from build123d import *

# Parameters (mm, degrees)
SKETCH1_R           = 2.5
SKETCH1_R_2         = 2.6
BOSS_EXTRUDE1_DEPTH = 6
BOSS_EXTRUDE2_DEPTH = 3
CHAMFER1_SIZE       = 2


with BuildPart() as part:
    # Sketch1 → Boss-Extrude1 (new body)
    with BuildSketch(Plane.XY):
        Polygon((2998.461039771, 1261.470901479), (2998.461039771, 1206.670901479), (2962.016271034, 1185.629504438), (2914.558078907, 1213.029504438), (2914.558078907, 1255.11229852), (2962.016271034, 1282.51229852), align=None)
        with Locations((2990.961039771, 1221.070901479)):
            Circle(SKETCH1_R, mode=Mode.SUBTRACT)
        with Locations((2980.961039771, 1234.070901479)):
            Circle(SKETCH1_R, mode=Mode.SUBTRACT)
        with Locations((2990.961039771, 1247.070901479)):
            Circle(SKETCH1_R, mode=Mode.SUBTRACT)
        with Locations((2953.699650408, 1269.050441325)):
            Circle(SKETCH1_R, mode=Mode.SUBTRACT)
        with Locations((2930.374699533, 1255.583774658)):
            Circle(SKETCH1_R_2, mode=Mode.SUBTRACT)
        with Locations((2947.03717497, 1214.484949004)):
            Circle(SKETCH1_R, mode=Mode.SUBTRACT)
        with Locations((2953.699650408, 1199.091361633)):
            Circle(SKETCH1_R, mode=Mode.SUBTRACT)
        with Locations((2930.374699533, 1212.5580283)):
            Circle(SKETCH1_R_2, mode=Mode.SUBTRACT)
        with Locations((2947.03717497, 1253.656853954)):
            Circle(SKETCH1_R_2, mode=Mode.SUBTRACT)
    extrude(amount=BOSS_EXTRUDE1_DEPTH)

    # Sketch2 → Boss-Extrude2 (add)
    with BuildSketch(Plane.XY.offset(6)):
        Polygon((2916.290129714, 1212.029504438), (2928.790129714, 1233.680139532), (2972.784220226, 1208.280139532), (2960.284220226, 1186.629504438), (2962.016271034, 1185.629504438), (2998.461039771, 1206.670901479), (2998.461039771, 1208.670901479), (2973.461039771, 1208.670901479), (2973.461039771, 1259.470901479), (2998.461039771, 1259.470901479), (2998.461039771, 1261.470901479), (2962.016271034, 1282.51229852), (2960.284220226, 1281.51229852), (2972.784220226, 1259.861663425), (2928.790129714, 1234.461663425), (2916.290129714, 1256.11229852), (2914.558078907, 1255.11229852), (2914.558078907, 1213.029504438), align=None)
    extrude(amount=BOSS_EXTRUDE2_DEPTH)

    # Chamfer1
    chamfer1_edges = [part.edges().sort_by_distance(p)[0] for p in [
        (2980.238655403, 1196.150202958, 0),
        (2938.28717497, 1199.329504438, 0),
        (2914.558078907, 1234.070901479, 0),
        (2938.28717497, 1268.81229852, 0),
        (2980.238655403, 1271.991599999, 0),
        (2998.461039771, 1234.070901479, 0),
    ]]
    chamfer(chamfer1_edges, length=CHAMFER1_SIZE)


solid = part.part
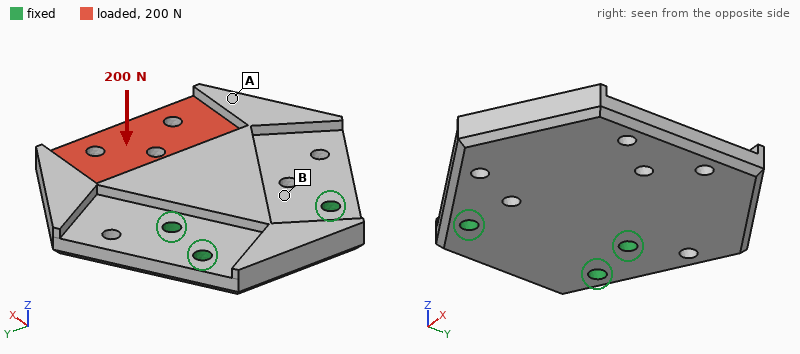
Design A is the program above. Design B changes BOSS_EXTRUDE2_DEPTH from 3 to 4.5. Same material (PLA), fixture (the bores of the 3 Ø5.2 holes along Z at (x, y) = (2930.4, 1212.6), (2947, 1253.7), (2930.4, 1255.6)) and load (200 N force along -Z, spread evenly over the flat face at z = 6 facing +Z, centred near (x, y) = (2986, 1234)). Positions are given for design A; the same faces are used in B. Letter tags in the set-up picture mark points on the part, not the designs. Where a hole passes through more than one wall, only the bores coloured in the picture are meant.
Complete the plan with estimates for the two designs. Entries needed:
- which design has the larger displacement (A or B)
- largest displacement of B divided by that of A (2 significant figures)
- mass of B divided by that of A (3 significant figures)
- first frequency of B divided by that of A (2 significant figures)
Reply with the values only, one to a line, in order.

A
0.86
1.08
1.0
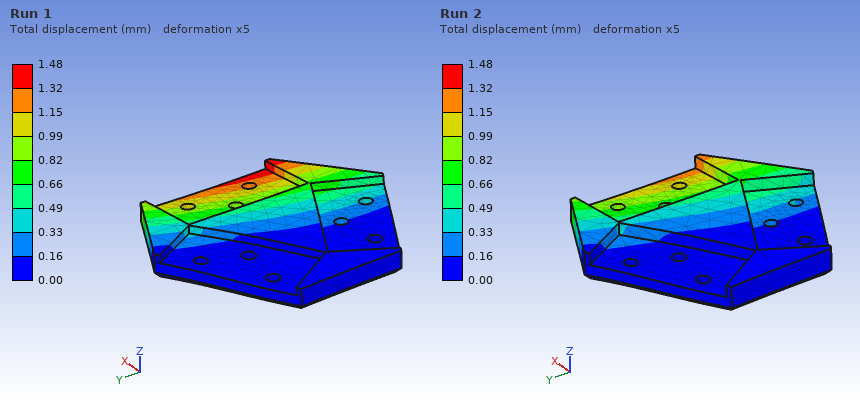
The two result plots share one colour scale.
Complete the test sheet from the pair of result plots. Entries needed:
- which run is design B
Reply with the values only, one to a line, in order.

Run 2
